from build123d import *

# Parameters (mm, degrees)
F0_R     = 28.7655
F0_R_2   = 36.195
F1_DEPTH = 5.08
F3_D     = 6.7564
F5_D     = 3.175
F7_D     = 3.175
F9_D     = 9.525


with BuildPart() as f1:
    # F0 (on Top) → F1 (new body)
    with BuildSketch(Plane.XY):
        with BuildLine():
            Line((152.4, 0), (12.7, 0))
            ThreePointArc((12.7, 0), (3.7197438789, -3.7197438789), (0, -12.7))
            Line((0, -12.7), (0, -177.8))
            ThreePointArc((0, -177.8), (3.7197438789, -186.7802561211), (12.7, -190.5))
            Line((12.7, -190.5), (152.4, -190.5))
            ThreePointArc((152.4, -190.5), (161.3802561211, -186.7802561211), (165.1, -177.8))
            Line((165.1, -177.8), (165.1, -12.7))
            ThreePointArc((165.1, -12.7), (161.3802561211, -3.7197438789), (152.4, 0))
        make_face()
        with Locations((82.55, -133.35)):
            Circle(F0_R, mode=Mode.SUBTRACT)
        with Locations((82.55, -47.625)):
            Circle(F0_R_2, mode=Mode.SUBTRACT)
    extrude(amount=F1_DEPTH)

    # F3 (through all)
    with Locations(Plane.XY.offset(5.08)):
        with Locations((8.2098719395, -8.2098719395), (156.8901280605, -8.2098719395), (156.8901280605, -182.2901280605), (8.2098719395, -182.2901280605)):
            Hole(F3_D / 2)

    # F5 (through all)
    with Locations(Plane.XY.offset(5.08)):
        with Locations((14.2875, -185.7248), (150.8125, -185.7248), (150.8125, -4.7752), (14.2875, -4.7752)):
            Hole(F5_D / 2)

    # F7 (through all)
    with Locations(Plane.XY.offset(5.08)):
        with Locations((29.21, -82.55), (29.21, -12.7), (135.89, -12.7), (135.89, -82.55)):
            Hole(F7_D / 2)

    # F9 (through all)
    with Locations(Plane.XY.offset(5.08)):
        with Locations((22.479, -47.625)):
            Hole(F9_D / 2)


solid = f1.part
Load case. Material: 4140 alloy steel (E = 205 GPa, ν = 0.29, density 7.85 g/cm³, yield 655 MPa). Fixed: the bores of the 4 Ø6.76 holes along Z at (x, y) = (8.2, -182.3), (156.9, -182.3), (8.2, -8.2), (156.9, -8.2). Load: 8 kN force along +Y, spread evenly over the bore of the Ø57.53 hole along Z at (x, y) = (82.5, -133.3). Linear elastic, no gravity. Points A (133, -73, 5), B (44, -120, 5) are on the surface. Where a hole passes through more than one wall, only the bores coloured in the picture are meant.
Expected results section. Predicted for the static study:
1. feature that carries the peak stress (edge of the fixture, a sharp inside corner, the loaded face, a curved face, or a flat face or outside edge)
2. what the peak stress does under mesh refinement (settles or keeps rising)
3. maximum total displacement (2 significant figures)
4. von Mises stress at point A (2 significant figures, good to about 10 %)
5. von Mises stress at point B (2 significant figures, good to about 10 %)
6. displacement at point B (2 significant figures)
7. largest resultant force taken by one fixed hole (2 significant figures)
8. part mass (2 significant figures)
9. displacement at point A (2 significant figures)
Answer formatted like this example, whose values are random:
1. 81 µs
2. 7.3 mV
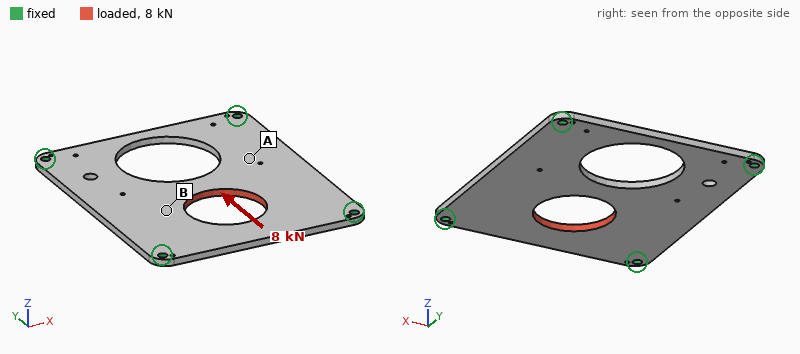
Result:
1. edge of the fixture
2. keeps rising
3. 12 µm
4. 7.4 MPa
5. 17 MPa
6. 6.0 µm
7. 2.5 kN
8. 970 g
9. 3.9 µm
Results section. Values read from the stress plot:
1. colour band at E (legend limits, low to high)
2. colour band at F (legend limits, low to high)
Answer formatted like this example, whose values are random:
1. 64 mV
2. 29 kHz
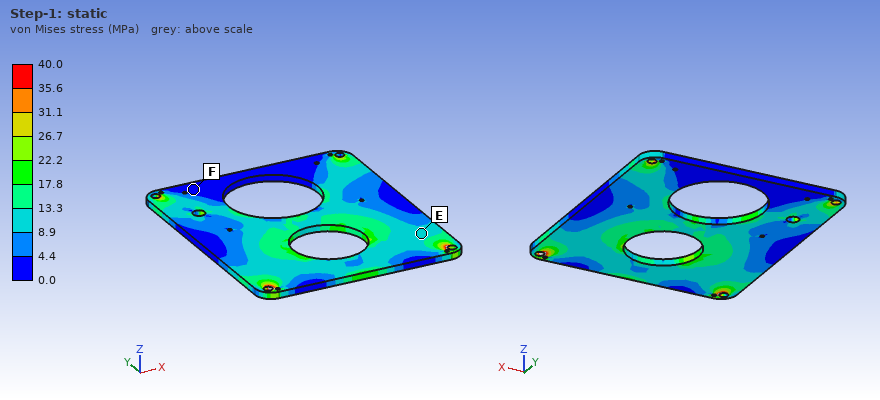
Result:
1. 8.9 to 13.3 MPa
2. 0.0 to 4.4 MPa
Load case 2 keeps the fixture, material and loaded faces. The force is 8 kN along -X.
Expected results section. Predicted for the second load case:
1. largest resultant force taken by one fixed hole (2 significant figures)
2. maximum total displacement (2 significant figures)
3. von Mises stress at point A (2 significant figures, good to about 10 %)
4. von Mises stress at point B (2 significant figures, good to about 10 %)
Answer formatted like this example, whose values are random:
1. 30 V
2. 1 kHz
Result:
1. 3.4 kN
2. 11 µm
3. 7.1 MPa
4. 7.4 MPa
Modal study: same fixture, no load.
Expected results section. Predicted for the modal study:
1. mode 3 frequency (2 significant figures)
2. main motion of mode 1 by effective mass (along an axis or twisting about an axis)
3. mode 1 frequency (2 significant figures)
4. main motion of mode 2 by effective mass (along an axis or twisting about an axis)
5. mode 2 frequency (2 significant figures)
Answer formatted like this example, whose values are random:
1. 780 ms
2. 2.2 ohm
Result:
1. 1200 Hz
2. along Z
3. 630 Hz
4. twisting about Y
5. 950 Hz
